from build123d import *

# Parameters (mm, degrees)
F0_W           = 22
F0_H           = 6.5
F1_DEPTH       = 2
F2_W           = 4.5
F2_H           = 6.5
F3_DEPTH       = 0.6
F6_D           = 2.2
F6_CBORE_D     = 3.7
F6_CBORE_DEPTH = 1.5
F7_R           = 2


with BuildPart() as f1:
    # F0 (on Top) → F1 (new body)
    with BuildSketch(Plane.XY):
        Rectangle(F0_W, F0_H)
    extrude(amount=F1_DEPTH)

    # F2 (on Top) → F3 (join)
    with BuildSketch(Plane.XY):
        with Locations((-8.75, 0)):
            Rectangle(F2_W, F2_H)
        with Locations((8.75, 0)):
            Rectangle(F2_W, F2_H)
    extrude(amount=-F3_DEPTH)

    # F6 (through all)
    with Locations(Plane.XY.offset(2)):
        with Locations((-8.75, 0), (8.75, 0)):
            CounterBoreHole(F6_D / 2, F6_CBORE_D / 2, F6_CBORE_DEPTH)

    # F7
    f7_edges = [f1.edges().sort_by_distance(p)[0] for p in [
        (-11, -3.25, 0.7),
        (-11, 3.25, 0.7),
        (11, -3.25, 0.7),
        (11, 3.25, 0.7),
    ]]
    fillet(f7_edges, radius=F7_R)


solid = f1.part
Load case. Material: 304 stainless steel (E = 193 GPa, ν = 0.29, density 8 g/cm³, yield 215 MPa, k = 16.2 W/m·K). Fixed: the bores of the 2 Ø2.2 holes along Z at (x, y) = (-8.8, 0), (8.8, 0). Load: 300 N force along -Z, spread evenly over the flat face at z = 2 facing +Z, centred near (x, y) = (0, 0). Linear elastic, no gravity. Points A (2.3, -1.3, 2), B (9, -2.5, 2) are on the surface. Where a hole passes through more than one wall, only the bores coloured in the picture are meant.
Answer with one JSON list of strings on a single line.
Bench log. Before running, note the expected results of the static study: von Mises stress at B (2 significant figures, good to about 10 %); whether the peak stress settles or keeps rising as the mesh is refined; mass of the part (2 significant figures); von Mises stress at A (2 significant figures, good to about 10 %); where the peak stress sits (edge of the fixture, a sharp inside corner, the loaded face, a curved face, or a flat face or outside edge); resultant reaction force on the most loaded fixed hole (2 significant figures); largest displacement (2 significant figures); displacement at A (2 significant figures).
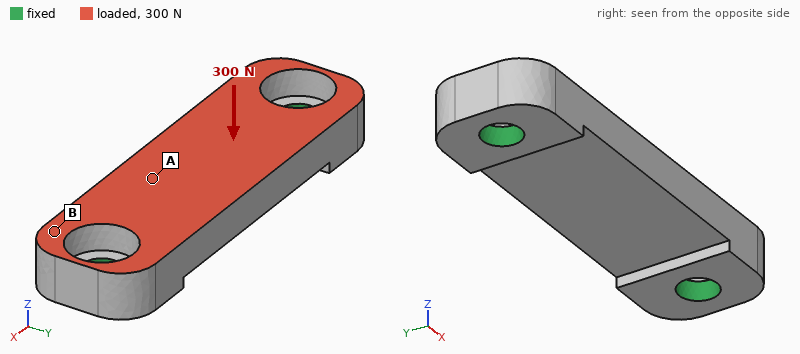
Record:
["19 MPa", "keeps rising", "2.2 g", "45 MPa", "edge of the fixture", "210 N", "5.4 µm", "4.5 µm"]
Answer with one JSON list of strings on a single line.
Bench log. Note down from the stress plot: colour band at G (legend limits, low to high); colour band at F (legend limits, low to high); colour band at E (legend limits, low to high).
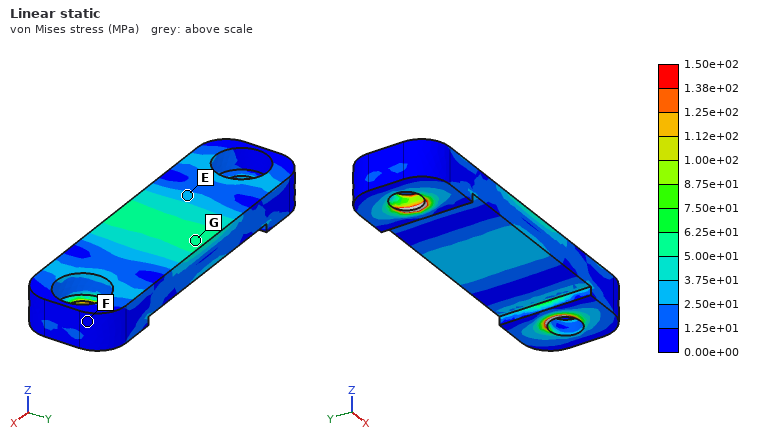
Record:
["5.00e+01 to 6.25e+01 MPa", "0.00e+00 to 1.25e+01 MPa", "2.50e+01 to 3.75e+01 MPa"]
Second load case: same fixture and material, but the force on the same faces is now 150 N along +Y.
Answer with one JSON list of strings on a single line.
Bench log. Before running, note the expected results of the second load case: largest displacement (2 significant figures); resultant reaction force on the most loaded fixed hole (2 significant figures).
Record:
["2.7 µm", "75 N"]
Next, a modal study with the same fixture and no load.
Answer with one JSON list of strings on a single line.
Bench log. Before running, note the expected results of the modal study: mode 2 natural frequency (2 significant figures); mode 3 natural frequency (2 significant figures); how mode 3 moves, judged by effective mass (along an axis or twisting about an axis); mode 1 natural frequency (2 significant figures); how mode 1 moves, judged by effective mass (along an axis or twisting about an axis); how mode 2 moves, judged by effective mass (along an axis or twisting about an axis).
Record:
["38 kHz", "54 kHz", "along Y", "31 kHz", "along Z", "along Y"]
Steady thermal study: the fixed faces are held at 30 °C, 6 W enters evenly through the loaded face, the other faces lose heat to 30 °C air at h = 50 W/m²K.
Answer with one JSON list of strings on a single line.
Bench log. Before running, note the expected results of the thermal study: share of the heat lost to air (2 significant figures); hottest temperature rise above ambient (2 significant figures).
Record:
["8.9 %", "68 K"]
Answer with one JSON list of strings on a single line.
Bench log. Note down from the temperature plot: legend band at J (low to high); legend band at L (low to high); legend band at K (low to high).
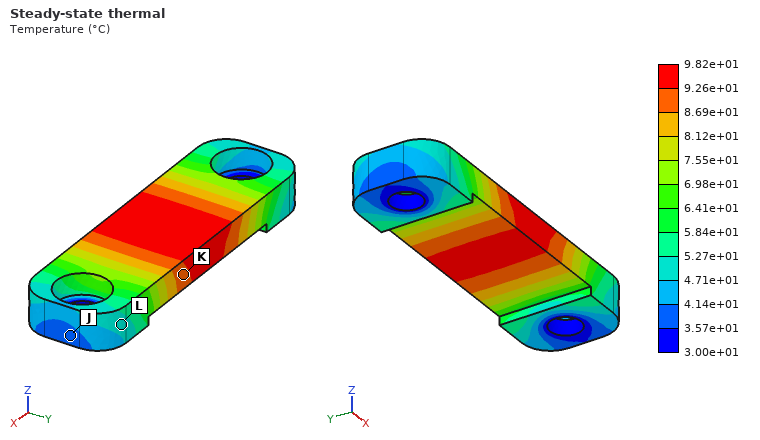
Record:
["3.57e+01 to 4.14e+01 °C", "4.71e+01 to 5.27e+01 °C", "8.69e+01 to 9.26e+01 °C"]
